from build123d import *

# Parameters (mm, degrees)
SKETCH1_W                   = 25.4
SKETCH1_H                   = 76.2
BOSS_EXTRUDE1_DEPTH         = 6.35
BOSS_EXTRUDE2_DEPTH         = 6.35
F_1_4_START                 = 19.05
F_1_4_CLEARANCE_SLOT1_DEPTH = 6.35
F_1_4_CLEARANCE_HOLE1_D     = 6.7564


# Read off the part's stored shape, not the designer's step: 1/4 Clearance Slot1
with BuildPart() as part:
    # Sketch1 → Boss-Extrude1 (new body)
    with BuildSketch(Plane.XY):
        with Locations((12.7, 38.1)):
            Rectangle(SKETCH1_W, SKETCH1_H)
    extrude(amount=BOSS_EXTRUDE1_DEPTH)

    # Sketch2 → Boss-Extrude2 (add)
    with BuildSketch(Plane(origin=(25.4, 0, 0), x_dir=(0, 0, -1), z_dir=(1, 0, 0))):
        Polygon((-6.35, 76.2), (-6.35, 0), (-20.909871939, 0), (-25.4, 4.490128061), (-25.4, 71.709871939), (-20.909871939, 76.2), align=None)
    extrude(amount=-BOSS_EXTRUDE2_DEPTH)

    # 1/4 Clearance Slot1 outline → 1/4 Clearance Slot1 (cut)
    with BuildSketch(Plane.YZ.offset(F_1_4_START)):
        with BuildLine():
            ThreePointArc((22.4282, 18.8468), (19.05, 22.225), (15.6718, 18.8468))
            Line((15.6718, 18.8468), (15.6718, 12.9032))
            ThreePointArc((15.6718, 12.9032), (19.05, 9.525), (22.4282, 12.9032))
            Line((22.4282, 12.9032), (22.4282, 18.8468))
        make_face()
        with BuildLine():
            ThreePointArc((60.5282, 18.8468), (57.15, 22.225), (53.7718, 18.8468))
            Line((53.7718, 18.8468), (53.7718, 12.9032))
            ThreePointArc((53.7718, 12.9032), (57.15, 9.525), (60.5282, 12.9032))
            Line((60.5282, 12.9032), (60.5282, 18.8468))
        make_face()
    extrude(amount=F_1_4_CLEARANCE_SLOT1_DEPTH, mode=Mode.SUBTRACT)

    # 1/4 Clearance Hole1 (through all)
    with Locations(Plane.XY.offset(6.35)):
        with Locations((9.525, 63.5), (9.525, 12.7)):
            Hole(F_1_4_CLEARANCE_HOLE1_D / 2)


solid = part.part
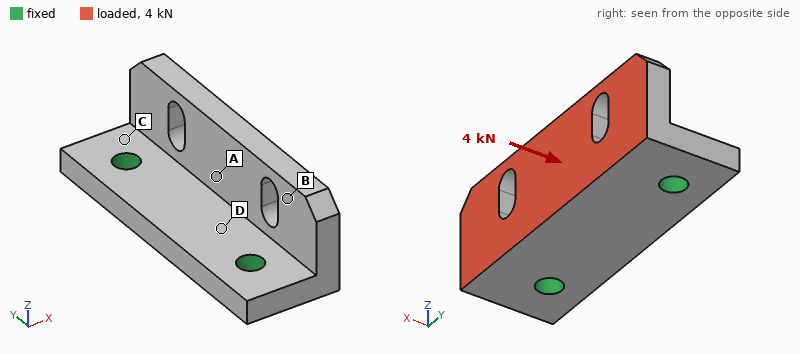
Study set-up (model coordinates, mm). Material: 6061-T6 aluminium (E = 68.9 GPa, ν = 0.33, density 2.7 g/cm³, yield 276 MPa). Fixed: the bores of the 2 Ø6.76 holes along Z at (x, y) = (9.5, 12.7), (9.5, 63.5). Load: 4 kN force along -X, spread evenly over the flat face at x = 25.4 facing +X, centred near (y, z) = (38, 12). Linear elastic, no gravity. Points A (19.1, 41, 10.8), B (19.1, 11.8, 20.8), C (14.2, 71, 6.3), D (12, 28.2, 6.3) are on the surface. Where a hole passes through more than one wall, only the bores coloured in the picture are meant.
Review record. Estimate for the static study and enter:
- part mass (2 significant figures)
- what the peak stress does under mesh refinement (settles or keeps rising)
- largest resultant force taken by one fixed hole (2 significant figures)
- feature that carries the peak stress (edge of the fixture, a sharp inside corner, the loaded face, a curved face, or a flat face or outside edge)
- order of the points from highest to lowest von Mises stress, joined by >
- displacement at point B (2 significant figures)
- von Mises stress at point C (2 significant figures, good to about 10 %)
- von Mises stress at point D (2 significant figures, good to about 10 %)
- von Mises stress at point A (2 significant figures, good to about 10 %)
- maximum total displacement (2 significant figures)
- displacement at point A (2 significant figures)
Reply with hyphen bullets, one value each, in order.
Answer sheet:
- 54 g
- keeps rising
- 2.0 kN
- edge of the fixture
- C > D > A > B
- 0.10 mm
- 66 MPa
- 43 MPa
- 31 MPa
- 0.15 mm
- 0.049 mm
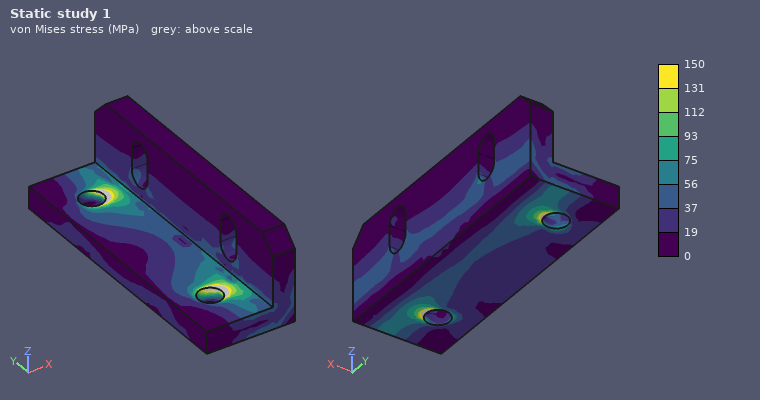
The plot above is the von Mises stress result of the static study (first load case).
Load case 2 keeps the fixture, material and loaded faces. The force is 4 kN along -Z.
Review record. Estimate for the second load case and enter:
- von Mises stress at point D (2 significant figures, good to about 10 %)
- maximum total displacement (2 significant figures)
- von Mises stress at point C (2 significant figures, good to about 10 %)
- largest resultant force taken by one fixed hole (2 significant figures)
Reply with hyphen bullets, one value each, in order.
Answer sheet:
- 38 MPa
- 0.14 mm
- 73 MPa
- 2.0 kN
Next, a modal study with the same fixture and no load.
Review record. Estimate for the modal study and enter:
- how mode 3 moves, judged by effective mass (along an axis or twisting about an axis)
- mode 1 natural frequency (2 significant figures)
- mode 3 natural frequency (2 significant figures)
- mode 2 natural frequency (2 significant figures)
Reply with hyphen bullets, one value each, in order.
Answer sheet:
- along Z
- 5400 Hz
- 12 kHz
- 7900 Hz
